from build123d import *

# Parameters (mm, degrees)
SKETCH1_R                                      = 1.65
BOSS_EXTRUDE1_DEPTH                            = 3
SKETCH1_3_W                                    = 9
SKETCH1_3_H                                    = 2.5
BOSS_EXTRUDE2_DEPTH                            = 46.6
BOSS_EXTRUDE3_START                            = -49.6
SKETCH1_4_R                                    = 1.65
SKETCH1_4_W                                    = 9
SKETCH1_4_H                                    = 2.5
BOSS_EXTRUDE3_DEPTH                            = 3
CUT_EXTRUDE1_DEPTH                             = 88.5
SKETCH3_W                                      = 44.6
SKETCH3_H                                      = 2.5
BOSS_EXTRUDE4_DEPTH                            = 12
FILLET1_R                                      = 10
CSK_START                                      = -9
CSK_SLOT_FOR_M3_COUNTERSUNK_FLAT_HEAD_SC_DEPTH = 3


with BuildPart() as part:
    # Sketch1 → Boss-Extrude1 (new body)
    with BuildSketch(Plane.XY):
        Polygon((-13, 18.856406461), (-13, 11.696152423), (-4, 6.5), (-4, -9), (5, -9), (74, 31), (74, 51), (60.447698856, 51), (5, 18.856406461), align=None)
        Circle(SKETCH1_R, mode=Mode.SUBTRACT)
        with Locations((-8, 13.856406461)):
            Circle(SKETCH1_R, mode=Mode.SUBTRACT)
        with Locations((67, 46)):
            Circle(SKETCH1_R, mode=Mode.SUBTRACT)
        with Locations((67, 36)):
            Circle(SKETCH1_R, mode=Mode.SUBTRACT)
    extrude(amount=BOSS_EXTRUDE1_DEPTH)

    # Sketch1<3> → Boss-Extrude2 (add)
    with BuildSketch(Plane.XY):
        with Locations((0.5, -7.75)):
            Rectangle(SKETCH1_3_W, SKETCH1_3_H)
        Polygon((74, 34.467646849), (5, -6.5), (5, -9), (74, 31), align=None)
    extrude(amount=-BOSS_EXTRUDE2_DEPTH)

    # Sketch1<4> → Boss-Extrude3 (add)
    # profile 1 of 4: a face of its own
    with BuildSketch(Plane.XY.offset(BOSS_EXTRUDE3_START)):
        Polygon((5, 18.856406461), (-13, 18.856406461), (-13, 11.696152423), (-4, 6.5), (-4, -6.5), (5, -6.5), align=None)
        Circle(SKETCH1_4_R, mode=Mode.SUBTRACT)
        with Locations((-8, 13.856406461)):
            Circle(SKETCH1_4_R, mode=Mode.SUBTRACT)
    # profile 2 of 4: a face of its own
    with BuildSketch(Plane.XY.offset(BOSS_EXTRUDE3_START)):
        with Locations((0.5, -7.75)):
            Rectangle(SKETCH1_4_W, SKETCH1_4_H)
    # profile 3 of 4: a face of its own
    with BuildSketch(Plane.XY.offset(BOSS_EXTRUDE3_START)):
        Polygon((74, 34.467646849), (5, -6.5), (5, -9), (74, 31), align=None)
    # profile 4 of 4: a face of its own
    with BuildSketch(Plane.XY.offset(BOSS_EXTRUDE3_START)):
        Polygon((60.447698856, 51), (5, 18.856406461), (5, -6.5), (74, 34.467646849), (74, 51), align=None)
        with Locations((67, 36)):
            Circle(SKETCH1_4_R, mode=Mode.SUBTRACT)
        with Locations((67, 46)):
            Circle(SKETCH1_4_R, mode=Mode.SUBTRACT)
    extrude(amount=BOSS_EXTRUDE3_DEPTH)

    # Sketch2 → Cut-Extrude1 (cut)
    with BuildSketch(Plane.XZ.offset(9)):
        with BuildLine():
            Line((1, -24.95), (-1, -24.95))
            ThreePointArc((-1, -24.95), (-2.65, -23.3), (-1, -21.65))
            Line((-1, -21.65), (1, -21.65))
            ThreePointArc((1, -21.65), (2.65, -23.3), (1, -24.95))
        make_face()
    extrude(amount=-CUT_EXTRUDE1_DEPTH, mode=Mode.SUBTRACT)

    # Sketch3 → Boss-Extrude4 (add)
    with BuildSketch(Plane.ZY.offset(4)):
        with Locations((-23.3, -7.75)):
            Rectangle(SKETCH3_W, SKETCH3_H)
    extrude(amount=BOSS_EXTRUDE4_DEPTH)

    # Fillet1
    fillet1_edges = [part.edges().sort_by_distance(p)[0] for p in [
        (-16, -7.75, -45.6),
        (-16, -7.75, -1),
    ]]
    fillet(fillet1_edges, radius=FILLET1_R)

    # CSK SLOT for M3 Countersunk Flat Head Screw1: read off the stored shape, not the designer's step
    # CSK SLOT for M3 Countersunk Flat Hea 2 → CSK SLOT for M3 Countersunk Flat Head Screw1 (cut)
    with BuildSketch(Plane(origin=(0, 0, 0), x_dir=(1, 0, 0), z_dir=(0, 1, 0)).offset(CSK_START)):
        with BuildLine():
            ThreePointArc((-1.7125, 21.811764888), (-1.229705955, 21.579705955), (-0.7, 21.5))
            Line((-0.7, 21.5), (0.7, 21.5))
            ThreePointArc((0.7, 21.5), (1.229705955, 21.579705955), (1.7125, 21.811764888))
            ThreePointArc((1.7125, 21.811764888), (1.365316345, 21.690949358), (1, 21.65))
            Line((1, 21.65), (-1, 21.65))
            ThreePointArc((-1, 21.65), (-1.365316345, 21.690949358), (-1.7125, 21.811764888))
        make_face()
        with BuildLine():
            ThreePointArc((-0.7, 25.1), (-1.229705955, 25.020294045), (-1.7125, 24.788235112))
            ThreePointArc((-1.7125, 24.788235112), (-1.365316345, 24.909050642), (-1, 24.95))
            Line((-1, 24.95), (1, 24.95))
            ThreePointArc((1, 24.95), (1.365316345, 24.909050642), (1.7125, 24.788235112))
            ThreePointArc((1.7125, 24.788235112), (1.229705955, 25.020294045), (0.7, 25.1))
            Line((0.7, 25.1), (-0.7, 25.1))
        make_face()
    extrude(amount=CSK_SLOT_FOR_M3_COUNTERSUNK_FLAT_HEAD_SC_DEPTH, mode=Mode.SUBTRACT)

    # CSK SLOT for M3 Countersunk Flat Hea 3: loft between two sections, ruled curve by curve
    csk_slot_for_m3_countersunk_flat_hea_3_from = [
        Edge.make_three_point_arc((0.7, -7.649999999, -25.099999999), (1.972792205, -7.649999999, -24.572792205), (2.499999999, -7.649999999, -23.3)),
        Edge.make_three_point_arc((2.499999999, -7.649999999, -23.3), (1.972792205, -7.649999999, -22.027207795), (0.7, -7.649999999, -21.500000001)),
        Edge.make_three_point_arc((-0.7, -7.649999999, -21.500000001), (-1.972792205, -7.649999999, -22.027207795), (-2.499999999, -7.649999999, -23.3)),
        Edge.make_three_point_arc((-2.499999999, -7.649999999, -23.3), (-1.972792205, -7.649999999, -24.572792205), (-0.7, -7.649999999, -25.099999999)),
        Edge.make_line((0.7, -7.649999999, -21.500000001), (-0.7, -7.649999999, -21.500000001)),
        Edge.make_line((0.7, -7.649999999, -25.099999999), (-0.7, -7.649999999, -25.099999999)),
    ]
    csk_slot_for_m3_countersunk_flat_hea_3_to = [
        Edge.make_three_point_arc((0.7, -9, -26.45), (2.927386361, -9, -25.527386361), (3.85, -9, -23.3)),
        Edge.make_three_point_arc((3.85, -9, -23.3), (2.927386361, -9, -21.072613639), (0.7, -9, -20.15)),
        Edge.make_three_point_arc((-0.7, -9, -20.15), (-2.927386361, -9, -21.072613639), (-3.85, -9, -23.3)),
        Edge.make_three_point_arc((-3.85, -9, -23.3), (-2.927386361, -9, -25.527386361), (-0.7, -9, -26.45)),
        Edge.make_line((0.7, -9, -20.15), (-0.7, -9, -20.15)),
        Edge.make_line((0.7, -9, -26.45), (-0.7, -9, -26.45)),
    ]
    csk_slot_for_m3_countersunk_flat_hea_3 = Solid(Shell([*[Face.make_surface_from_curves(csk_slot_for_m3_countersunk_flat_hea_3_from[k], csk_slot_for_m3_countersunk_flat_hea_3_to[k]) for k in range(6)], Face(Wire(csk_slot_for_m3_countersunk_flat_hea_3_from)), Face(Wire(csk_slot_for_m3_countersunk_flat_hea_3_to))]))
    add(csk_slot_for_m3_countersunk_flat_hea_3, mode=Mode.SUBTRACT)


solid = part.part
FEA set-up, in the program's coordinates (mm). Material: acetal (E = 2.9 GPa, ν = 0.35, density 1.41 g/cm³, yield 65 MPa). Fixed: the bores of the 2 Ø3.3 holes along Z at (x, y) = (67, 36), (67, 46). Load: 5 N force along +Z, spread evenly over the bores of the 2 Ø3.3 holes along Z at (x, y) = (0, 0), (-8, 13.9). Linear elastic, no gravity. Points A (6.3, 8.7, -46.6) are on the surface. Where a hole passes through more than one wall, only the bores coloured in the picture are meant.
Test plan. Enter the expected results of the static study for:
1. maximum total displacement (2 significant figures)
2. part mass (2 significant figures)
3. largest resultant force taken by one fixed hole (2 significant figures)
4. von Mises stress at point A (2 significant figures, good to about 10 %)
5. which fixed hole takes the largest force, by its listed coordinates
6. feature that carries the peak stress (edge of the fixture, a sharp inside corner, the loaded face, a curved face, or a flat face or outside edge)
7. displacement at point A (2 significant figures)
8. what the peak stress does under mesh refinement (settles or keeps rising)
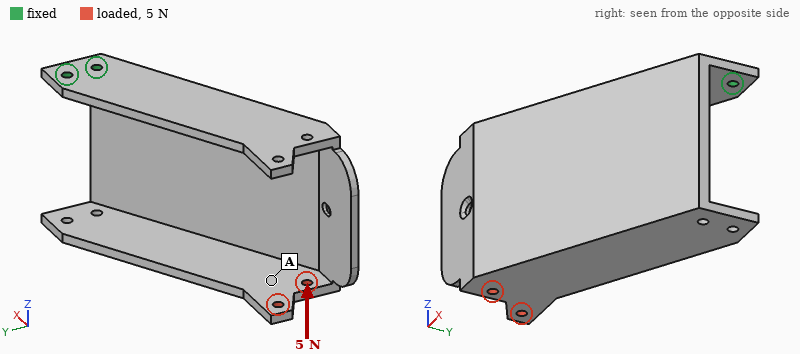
1.3 mm
35 g
10 N
1.0 MPa
(67, 36)
edge of the fixture
0.97 mm
keeps rising
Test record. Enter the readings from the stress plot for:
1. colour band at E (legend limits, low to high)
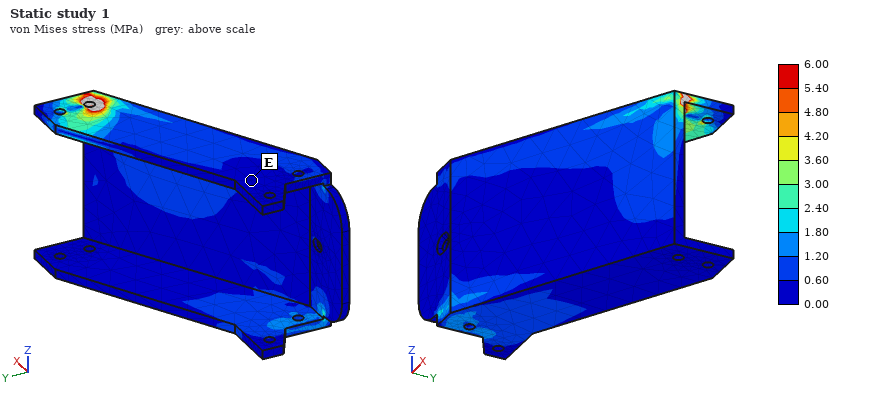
0.00 to 0.60 MPa
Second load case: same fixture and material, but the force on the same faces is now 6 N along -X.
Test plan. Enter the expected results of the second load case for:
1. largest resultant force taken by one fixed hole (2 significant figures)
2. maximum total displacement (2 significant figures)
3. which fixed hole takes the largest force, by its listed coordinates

18 N
1.3 mm
(67, 36)
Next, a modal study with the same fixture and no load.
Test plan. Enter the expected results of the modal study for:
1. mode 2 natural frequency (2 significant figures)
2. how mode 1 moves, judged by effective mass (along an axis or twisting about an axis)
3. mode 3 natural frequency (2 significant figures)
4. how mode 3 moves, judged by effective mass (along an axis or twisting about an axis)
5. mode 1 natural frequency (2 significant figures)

90 Hz
along Y
210 Hz
twisting about Z
77 Hz
